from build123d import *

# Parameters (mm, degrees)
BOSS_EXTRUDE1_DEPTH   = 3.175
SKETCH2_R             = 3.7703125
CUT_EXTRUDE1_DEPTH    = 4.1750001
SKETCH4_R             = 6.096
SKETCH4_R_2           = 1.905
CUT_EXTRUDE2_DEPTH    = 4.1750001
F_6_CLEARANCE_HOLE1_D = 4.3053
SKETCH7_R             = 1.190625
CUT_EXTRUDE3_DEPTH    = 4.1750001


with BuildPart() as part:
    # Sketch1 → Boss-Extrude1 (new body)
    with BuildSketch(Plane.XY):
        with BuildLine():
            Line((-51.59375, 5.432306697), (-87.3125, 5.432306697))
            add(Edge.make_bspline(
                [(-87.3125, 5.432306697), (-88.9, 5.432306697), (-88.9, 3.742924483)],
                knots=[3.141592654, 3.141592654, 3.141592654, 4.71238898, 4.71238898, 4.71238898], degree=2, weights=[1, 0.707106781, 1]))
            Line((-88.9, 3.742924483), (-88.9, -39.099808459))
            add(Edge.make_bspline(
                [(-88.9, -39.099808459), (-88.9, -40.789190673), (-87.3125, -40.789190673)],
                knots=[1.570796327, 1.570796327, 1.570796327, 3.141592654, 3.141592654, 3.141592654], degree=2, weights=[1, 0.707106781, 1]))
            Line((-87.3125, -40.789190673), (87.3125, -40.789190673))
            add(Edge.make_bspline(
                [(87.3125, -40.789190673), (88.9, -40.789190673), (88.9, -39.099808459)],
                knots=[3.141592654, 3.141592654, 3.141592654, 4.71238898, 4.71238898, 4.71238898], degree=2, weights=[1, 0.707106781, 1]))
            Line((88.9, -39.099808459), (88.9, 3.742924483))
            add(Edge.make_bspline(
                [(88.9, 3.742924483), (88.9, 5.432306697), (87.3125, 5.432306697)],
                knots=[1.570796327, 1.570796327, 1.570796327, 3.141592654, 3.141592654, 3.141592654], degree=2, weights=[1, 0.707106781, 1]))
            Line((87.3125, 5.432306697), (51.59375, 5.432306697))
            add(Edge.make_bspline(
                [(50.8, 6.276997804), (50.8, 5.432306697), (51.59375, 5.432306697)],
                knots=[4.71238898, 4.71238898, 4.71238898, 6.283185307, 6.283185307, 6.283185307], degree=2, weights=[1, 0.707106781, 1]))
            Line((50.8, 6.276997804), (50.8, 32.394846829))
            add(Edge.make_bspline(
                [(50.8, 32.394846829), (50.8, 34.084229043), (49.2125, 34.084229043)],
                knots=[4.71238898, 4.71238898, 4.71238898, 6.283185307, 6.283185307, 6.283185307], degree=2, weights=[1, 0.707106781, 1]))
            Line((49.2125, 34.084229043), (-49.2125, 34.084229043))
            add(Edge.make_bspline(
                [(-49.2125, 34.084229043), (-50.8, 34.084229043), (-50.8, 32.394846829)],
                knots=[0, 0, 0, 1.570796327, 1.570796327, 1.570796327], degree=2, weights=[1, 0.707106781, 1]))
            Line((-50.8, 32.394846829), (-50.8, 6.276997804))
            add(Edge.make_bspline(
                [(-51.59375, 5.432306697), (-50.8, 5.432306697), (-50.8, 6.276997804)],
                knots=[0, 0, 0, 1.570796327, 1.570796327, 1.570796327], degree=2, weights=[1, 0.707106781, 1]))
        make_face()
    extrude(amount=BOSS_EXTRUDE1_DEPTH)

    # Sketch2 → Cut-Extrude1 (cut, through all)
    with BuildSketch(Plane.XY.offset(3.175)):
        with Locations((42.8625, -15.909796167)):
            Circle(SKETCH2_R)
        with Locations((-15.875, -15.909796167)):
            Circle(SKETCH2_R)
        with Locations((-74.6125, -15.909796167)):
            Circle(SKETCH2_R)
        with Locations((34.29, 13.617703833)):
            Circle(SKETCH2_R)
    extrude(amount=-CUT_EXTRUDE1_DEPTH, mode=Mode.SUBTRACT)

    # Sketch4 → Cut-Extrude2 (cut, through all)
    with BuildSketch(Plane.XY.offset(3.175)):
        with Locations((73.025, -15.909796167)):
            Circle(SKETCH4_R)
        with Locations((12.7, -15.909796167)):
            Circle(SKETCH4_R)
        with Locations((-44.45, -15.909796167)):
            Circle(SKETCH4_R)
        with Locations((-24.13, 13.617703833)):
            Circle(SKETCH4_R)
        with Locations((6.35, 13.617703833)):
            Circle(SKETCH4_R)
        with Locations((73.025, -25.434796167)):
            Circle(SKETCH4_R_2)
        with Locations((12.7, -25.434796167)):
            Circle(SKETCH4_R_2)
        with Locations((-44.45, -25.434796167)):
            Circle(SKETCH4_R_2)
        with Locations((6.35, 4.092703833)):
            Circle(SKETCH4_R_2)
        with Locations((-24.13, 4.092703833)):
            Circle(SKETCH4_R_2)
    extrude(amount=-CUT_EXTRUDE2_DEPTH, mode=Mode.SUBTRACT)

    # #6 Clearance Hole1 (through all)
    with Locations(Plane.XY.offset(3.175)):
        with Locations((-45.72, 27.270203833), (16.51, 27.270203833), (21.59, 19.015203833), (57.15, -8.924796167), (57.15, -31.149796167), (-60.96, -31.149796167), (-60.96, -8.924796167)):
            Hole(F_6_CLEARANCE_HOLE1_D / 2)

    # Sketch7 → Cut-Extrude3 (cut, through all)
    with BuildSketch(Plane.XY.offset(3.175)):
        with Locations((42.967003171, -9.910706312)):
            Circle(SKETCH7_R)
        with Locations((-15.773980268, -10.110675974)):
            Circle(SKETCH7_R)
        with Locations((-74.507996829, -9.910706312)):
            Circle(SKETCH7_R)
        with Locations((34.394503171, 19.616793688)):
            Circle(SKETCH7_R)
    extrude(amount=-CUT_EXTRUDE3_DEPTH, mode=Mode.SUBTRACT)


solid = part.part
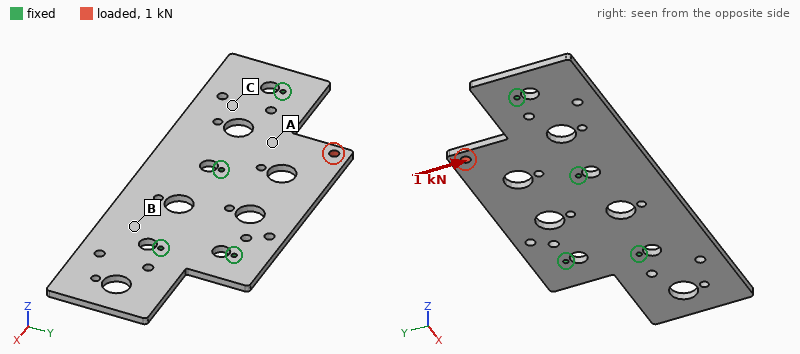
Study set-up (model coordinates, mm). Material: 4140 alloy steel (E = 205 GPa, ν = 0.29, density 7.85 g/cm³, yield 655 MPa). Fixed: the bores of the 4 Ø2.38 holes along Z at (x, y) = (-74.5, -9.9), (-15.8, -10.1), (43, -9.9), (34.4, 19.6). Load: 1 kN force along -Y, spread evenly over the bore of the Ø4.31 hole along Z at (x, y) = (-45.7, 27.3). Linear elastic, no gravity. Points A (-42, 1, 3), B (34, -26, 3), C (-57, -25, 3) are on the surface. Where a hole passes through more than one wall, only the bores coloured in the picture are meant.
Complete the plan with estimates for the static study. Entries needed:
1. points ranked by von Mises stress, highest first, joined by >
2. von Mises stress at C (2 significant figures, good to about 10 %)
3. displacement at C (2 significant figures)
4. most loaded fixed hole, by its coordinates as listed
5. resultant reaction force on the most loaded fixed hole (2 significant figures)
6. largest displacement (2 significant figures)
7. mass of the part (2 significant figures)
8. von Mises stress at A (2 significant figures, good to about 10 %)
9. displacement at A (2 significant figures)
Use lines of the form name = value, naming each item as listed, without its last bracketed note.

points ranked by von Mises stress, highest first, joined by > = A > C > B
von Mises stress at C = 5.4 MPa
displacement at C = 1.6 µm
most loaded fixed hole, by its coordinates as listed = (-15.8, -10.1)
resultant reaction force on the most loaded fixed hole = 670 N
largest displacement = 7.1 µm
mass of the part = 250 g
von Mises stress at A = 10 MPa
displacement at A = 2.9 µm
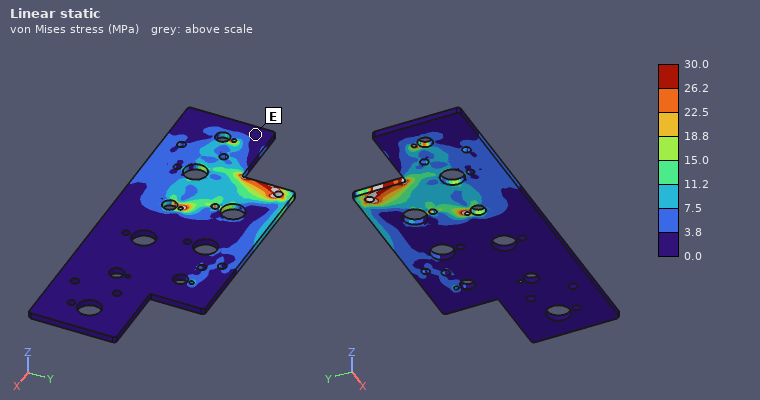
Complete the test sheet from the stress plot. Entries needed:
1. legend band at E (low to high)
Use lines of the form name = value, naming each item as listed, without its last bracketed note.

legend band at E = 0.0 to 3.8 MPa
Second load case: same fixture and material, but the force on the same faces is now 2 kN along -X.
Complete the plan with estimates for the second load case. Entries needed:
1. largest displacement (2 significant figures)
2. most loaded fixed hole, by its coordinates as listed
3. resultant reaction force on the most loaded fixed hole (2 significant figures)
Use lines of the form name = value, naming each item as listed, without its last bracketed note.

largest displacement = 13 µm
most loaded fixed hole, by its coordinates as listed = (34.4, 19.6)
resultant reaction force on the most loaded fixed hole = 800 N
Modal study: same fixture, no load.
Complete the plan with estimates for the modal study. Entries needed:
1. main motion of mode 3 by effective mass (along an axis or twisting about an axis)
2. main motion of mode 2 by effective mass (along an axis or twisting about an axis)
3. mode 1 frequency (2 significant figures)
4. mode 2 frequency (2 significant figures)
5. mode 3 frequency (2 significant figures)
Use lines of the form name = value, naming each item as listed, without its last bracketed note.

main motion of mode 3 by effective mass = along Z
main motion of mode 2 by effective mass = twisting about X
mode 1 frequency = 990 Hz
mode 2 frequency = 1300 Hz
mode 3 frequency = 1700 Hz
